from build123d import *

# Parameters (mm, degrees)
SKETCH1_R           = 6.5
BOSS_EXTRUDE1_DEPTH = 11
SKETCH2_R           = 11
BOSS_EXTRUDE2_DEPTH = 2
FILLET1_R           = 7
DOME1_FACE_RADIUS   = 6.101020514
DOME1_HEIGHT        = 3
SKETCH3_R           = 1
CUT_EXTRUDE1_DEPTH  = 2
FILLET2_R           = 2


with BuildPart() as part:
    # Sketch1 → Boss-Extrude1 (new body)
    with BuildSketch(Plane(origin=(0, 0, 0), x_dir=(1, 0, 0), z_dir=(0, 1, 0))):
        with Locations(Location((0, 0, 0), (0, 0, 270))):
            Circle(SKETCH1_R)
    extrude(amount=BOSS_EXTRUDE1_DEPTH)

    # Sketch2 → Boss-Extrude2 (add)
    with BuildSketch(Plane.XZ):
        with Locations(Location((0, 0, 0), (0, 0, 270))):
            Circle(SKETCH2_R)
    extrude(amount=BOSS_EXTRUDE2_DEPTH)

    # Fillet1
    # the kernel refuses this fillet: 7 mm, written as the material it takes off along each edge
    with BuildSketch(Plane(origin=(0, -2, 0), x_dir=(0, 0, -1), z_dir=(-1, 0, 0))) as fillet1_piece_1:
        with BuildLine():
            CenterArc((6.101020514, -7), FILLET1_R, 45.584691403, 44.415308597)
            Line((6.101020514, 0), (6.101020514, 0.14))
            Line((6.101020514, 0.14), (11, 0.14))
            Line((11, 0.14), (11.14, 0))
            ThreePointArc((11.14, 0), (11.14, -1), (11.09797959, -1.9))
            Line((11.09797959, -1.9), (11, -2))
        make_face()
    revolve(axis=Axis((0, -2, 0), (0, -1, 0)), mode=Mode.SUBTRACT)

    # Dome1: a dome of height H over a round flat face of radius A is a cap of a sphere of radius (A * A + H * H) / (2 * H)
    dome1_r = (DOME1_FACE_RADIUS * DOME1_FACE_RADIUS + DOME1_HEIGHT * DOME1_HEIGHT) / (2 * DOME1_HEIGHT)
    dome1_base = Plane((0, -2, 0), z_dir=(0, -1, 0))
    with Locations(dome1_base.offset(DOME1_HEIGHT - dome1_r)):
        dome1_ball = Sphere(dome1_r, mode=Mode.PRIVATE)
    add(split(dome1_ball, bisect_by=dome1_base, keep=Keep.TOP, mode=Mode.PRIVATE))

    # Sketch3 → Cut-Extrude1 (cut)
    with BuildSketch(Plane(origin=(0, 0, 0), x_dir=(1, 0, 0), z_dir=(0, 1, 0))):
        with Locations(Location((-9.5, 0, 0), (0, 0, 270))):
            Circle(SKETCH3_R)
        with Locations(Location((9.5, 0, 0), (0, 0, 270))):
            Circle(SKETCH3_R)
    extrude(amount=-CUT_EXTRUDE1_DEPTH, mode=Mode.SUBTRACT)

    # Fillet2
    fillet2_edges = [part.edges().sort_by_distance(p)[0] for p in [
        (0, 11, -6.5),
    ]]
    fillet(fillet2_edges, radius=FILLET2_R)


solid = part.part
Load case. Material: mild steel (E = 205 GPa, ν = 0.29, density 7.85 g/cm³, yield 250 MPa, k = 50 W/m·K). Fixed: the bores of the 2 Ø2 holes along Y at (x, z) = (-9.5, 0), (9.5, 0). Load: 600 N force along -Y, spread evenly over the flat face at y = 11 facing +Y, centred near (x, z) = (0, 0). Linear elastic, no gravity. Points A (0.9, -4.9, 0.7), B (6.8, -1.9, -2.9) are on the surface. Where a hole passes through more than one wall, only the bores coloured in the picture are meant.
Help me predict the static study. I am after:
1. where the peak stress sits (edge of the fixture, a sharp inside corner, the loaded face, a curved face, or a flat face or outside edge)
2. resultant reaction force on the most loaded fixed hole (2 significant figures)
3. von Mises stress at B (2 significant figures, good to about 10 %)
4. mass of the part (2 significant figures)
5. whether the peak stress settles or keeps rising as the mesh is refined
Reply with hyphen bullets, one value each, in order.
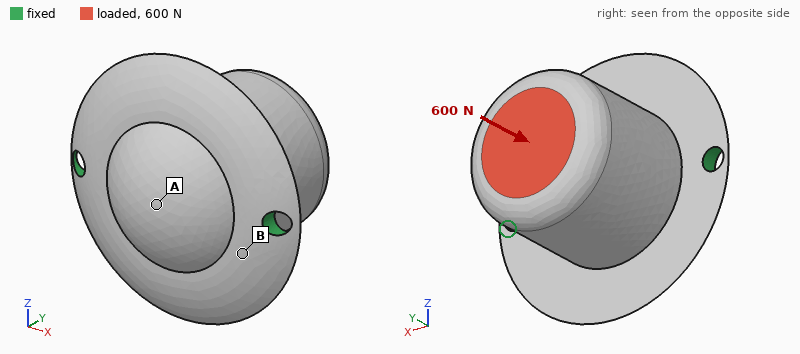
- edge of the fixture
- 300 N
- 46 MPa
- 17 g
- keeps rising
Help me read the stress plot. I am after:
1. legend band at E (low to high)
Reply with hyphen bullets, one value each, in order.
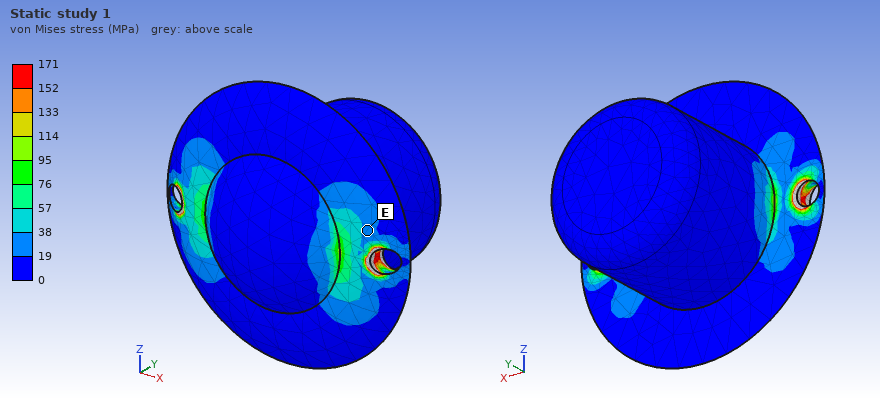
- 19 to 38 MPa
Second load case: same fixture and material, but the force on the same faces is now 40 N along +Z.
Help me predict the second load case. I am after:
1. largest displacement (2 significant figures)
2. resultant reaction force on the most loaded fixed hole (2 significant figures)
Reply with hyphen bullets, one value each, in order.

- 11 µm
- 20 N
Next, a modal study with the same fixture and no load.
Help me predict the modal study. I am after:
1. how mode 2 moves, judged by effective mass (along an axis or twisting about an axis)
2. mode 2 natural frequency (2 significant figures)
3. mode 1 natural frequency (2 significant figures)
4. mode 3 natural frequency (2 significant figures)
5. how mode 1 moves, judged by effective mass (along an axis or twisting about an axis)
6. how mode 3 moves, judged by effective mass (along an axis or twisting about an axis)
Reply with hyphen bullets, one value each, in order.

- along Y
- 16 kHz
- 4300 Hz
- 17 kHz
- along Z
- along X
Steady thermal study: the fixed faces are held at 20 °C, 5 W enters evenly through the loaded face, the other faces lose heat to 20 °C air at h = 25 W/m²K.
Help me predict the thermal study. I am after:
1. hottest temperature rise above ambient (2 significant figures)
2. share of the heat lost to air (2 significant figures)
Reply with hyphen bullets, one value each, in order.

- 25 K
- 8.9 %
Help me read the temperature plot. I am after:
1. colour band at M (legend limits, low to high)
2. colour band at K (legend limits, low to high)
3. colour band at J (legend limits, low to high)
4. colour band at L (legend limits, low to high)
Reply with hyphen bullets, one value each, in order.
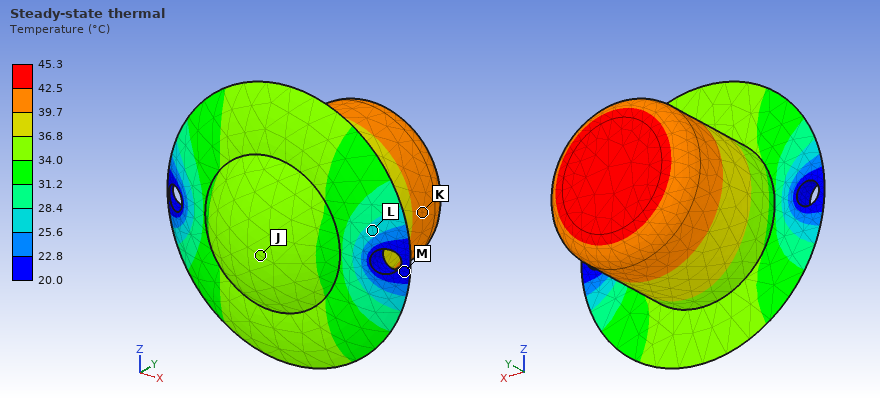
- 20.0 to 22.8 °C
- 39.7 to 42.5 °C
- 34.0 to 36.8 °C
- 25.6 to 28.4 °C
